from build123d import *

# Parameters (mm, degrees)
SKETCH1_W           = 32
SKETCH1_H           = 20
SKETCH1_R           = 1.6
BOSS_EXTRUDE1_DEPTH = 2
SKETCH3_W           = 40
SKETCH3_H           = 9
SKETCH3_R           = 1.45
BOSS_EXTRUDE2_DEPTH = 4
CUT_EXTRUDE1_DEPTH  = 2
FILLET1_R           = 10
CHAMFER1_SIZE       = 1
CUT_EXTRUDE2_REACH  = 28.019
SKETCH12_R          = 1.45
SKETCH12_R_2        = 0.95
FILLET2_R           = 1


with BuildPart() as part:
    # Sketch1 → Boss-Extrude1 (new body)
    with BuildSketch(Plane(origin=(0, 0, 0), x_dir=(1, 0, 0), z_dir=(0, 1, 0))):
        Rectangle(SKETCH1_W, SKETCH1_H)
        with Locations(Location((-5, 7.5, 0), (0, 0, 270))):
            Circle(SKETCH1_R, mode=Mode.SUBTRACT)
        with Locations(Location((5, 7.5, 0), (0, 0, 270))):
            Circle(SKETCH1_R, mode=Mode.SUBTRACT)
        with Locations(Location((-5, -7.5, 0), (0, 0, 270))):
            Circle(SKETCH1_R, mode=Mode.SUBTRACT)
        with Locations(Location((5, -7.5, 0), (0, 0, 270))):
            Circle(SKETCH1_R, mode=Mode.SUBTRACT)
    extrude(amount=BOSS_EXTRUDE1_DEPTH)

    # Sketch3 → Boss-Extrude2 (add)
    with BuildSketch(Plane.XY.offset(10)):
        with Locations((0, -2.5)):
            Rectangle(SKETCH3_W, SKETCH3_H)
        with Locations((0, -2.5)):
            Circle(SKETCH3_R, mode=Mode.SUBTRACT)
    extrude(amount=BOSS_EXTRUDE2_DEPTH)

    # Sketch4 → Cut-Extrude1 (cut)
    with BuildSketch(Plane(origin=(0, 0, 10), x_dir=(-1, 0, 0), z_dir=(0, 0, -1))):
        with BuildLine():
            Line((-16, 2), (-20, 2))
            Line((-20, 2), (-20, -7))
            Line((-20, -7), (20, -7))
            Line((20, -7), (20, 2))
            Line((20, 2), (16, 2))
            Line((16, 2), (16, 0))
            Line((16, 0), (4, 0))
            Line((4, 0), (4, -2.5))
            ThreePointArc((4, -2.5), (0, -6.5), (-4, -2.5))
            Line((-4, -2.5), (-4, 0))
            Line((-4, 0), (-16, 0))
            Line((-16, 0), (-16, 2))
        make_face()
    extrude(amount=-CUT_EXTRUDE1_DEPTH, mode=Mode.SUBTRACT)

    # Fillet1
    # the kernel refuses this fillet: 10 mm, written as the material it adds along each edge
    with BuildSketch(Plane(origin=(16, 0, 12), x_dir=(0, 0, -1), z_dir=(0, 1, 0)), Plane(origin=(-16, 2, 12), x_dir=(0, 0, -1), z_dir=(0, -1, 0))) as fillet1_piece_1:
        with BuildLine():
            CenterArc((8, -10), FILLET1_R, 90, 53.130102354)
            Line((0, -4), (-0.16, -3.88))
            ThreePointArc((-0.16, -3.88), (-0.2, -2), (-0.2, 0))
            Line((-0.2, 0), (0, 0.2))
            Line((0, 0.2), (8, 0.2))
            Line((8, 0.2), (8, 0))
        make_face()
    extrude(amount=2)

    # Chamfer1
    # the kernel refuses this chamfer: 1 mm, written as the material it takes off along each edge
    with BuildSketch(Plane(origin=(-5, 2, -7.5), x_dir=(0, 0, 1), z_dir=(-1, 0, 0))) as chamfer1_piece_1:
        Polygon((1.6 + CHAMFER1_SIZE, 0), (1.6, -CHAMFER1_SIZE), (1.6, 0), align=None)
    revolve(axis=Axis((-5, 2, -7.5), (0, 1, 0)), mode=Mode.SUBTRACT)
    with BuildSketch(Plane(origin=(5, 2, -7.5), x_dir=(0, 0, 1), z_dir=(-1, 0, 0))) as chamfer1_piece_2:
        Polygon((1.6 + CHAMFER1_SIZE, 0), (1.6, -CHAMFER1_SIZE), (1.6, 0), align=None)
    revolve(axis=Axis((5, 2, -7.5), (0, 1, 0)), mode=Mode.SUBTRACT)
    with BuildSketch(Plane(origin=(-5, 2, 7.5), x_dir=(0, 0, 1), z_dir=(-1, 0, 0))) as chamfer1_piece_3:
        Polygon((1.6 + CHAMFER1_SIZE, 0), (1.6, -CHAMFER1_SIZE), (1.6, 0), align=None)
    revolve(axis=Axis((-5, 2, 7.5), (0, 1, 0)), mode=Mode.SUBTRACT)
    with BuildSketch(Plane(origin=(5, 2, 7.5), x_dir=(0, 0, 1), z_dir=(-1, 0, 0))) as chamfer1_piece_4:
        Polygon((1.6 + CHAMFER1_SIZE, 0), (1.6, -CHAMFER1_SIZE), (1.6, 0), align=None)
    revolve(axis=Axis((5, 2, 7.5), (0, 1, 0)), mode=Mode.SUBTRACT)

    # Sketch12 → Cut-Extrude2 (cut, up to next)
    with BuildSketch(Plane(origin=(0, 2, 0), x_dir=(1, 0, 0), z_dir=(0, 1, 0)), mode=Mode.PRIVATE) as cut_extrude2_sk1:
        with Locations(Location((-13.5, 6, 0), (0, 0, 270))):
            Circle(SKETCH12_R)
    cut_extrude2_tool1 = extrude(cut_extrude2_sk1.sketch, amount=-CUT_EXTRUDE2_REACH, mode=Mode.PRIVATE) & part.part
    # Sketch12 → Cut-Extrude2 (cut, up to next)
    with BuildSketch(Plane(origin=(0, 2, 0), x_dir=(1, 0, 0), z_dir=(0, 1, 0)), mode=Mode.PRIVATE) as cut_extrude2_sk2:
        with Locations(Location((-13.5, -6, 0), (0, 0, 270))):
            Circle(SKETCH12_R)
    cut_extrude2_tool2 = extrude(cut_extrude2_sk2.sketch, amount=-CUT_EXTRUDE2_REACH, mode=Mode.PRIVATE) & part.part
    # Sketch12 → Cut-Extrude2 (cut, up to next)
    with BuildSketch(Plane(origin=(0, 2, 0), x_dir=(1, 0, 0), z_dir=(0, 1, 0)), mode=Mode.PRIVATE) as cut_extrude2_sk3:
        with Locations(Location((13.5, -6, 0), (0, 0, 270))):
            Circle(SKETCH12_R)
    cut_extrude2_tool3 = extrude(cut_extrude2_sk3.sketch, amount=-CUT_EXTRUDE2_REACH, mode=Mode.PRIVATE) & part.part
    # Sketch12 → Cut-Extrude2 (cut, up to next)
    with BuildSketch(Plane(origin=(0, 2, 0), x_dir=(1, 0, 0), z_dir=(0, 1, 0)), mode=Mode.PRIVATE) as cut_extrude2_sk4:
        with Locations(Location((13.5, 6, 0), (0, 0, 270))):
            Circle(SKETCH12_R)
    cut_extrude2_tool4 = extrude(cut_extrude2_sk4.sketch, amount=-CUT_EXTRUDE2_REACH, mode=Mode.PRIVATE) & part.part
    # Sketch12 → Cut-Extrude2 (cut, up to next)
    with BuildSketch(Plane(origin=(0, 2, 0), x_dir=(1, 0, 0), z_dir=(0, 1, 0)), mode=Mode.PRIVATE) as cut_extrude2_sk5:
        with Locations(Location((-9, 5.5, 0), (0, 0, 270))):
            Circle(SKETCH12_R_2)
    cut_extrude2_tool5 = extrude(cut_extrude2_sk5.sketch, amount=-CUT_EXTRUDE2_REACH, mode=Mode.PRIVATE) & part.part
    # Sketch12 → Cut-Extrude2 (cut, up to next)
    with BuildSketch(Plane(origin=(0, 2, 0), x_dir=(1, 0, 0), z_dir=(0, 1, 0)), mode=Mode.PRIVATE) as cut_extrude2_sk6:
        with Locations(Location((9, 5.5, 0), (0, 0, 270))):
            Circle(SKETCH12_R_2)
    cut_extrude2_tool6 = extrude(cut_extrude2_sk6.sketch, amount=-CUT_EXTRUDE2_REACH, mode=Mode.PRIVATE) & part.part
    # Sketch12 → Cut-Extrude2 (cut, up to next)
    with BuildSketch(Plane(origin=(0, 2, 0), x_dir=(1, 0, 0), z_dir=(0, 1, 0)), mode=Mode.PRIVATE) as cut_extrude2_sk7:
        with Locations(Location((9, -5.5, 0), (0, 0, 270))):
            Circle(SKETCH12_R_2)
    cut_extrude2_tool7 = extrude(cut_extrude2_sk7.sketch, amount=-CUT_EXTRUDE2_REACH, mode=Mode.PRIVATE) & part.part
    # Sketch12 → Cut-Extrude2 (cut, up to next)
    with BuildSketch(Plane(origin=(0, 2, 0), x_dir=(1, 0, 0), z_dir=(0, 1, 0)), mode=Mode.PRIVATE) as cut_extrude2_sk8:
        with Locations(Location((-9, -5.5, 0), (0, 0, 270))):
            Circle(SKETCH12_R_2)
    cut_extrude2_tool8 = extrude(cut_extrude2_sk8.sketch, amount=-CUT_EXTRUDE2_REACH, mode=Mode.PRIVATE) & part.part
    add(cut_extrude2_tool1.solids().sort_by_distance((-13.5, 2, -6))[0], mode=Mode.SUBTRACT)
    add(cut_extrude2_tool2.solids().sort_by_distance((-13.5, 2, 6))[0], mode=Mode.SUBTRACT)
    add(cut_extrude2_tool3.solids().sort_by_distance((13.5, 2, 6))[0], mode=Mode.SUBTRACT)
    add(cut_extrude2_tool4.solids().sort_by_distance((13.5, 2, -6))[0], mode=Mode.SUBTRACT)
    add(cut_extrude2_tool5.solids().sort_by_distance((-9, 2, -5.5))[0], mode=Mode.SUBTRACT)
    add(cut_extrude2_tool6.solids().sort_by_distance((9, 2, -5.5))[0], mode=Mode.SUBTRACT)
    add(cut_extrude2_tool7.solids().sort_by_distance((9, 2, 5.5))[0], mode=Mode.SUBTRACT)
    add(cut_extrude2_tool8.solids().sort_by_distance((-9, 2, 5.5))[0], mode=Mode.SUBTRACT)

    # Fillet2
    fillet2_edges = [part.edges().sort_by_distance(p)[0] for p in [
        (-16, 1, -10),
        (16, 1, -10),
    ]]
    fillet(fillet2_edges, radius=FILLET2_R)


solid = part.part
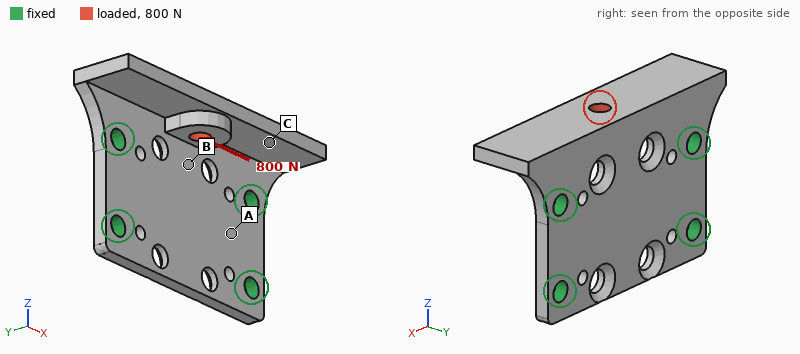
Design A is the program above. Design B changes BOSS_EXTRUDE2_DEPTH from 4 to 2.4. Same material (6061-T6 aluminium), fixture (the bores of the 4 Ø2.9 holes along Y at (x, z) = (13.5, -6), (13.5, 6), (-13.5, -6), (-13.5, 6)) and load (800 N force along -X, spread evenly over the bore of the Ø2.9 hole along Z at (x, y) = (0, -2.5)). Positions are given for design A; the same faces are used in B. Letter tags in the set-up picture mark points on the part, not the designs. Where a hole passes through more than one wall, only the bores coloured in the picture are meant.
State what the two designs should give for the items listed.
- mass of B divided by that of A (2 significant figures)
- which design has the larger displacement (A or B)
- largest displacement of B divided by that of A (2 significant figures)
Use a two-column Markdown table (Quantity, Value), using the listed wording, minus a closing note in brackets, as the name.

| Quantity | Value |
|---|---|
| mass of B divided by that of A | 0.73 |
| which design has the larger displacement | B |
| largest displacement of B divided by that of A | 1.1 |
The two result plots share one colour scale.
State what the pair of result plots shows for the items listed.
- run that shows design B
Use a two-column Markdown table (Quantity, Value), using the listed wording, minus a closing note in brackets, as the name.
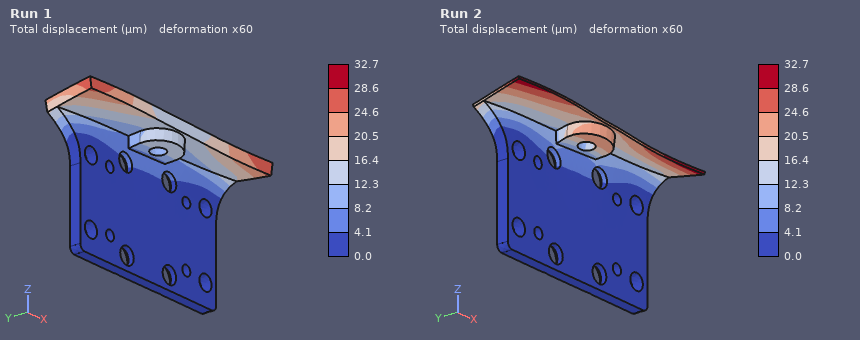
| Quantity | Value |
|---|---|
| run that shows design B | Run 2 |
